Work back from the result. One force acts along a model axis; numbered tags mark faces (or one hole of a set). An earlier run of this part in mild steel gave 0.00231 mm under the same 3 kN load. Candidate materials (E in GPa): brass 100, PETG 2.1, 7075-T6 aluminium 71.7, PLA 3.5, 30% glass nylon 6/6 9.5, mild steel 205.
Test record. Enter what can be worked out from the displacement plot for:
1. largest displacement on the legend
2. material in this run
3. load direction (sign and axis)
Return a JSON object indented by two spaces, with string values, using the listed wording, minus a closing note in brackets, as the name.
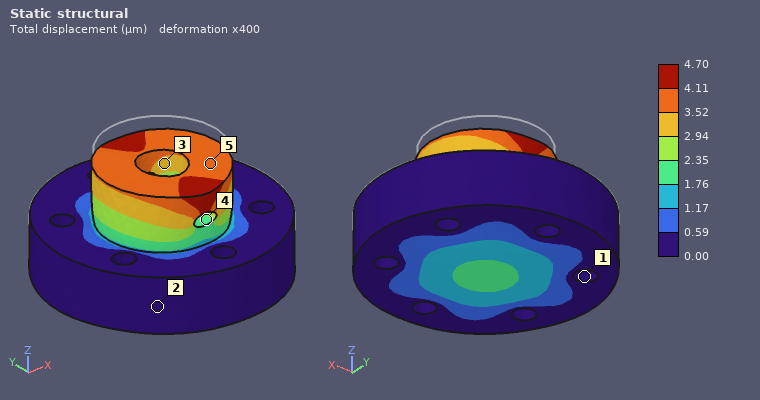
{
  "largest displacement on the legend": "4.70 µm",
  "material in this run": "brass",
  "load direction": "-Z"
}
